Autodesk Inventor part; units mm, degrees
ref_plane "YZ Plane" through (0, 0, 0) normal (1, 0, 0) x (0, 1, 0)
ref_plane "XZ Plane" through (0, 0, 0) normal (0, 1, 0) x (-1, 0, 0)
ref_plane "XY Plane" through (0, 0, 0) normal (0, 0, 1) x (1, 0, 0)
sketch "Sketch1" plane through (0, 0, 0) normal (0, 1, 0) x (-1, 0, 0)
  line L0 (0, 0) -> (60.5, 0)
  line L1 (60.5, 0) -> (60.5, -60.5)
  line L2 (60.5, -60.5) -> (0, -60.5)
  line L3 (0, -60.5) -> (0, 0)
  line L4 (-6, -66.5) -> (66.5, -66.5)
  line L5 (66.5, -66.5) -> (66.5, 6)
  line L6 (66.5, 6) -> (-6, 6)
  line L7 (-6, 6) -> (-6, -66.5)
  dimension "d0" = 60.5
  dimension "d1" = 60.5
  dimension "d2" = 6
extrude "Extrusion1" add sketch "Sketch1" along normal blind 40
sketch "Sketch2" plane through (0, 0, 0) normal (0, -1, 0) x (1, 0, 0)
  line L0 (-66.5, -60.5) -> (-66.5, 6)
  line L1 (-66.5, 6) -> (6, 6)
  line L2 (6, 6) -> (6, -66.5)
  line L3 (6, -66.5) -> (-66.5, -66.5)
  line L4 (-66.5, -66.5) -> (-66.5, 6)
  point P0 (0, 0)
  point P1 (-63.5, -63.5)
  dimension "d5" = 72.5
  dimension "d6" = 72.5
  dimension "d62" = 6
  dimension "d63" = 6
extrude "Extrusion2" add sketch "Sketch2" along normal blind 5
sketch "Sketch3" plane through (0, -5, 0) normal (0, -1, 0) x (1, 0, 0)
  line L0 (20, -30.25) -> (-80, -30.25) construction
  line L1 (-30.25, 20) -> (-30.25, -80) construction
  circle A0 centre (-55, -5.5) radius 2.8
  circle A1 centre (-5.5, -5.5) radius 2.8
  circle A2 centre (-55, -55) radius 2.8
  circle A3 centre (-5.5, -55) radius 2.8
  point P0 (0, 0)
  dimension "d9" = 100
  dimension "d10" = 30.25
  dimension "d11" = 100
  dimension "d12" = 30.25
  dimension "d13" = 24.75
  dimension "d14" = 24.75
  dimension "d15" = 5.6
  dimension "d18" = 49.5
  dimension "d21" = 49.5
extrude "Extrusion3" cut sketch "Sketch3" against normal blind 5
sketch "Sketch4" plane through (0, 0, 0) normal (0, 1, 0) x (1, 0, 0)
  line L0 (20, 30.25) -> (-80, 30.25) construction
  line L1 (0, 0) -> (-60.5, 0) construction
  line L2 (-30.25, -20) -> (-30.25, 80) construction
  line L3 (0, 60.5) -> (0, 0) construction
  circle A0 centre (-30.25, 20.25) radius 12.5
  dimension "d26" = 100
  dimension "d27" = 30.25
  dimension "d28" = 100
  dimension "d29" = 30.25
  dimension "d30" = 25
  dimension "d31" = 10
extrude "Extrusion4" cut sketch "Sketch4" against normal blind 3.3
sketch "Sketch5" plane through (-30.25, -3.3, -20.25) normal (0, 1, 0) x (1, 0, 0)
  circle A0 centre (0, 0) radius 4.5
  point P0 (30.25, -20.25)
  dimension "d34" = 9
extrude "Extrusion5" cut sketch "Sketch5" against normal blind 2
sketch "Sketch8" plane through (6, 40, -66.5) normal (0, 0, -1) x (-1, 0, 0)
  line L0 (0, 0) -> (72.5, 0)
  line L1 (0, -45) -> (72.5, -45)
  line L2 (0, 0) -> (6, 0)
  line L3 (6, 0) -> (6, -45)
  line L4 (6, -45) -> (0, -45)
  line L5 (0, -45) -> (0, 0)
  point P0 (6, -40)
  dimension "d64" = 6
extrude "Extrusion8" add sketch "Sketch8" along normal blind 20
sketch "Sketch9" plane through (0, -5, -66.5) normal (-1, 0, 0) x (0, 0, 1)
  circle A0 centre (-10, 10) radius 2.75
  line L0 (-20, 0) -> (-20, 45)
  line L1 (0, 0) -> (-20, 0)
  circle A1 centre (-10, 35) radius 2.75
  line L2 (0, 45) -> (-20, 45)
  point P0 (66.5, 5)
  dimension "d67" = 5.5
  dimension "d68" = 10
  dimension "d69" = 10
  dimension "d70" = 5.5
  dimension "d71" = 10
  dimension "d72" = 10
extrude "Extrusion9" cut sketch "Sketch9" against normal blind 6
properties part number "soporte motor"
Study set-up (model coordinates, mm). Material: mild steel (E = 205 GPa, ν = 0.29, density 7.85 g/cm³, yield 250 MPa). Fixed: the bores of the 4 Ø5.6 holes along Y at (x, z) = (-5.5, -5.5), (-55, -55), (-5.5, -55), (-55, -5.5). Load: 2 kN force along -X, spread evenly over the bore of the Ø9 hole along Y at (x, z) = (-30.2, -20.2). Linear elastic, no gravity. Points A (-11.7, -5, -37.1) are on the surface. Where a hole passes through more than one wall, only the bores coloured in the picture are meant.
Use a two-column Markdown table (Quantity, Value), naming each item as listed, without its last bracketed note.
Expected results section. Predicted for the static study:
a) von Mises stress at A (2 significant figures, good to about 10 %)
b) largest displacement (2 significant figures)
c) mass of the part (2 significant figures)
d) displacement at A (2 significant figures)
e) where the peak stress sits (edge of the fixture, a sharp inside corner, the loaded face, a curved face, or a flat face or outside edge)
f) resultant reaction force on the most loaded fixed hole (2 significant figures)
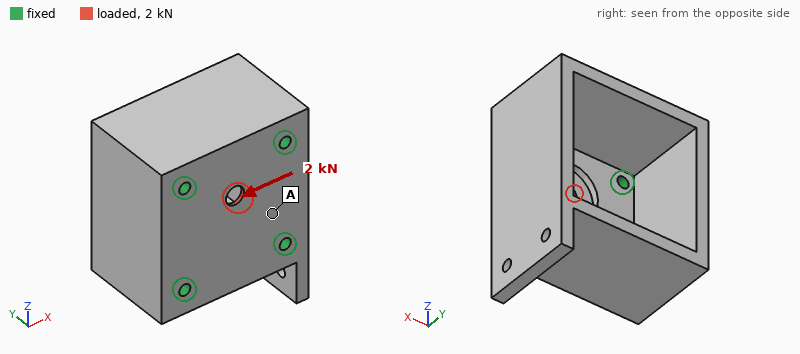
| Quantity | Value |
|---|---|
| von Mises stress at A | 5.7 MPa |
| largest displacement | 2.8 µm |
| mass of the part | 730 g |
| displacement at A | 0.57 µm |
| where the peak stress sits | the loaded face |
| resultant reaction force on the most loaded fixed hole | 680 N |
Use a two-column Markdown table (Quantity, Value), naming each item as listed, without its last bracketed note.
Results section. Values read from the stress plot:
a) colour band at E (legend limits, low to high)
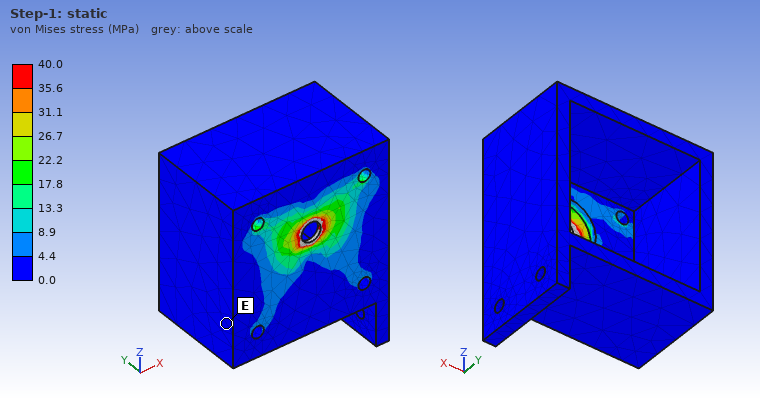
| Quantity | Value |
|---|---|
| colour band at E | 0.0 to 4.4 MPa |
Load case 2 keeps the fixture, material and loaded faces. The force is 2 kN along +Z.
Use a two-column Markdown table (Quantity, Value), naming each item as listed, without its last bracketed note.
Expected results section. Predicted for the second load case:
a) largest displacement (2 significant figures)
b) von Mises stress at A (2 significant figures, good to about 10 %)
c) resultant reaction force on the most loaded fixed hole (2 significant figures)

| Quantity | Value |
|---|---|
| largest displacement | 3.2 µm |
| von Mises stress at A | 6.0 MPa |
| resultant reaction force on the most loaded fixed hole | 600 N |
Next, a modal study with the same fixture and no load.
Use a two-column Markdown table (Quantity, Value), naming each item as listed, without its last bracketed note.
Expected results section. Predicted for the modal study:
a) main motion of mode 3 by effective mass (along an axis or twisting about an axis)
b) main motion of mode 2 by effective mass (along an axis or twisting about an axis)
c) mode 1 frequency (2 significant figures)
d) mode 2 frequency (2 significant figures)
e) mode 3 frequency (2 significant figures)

| Quantity | Value |
|---|---|
| main motion of mode 3 by effective mass | along X |
| main motion of mode 2 by effective mass | along Z |
| mode 1 frequency | 4800 Hz |
| mode 2 frequency | 5200 Hz |
| mode 3 frequency | 5500 Hz |
